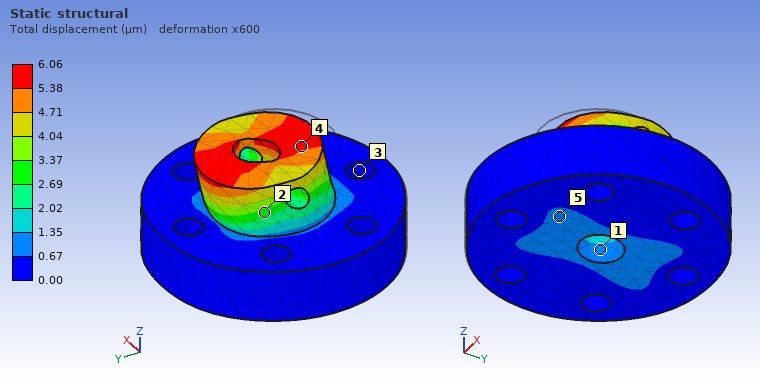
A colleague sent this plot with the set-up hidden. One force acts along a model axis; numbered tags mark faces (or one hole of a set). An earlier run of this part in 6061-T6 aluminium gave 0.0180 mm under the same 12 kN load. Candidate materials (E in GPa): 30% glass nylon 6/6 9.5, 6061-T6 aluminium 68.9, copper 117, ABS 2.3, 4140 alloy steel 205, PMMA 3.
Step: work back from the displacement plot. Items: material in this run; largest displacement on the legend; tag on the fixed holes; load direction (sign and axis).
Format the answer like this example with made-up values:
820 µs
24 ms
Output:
4140 alloy steel
6.06 µm
3
+Y
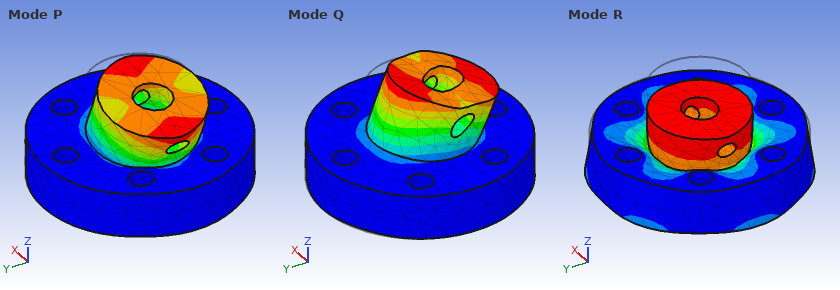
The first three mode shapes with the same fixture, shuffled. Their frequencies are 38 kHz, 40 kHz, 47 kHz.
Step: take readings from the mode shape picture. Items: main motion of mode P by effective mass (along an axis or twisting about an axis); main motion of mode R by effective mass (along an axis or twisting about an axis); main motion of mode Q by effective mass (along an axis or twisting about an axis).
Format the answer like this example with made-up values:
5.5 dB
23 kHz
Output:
along X
along Z
along Y
